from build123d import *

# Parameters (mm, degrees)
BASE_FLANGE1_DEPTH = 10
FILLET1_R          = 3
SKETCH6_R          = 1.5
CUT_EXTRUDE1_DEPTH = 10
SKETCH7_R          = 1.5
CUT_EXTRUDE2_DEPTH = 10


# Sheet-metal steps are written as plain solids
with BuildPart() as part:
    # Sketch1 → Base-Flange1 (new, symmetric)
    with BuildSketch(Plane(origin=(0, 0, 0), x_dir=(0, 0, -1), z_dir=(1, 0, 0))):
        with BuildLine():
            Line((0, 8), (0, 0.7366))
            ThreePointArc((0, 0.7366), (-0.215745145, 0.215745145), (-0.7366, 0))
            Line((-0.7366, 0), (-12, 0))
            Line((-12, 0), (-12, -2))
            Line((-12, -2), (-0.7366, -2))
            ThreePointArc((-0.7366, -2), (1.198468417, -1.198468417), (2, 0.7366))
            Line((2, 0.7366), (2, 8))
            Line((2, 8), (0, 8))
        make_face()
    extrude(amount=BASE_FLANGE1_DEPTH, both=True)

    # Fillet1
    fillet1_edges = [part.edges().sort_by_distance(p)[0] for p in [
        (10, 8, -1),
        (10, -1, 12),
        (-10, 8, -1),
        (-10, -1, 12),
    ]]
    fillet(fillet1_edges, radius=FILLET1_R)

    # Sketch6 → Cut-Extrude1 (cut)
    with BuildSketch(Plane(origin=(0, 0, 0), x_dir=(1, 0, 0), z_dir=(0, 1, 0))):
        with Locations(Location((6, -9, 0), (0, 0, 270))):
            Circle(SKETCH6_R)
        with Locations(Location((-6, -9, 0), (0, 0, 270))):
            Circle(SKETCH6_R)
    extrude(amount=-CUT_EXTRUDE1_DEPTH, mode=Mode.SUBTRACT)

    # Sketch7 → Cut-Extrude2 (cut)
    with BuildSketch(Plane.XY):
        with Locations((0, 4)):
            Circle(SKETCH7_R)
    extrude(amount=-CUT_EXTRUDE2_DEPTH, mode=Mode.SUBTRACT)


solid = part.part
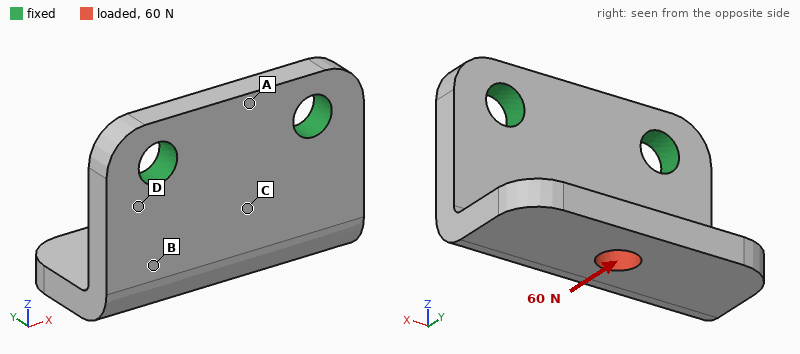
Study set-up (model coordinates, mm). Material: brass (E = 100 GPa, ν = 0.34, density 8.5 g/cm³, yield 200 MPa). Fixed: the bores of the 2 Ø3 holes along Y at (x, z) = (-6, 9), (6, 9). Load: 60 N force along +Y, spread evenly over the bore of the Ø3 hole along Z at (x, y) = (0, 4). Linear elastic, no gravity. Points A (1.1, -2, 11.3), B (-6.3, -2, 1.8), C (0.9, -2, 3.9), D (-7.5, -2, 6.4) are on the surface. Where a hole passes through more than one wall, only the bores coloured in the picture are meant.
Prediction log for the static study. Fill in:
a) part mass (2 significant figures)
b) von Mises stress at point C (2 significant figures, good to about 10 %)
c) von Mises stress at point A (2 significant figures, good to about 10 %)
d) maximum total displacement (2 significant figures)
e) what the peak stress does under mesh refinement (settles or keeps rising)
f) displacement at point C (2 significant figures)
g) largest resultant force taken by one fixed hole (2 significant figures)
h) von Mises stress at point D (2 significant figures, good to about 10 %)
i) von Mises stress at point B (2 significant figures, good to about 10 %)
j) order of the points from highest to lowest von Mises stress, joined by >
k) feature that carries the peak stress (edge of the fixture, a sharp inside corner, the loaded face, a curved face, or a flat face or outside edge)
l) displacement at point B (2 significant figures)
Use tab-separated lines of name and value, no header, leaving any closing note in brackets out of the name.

part mass	6.7 g
von Mises stress at point C	18 MPa
von Mises stress at point A	5.4 MPa
maximum total displacement	22 µm
what the peak stress does under mesh refinement	keeps rising
displacement at point C	4.4 µm
largest resultant force taken by one fixed hole	30 N
von Mises stress at point D	33 MPa
von Mises stress at point B	12 MPa
order of the points from highest to lowest von Mises stress, joined by >	D > C > B > A
feature that carries the peak stress	edge of the fixture
displacement at point B	7.2 µm
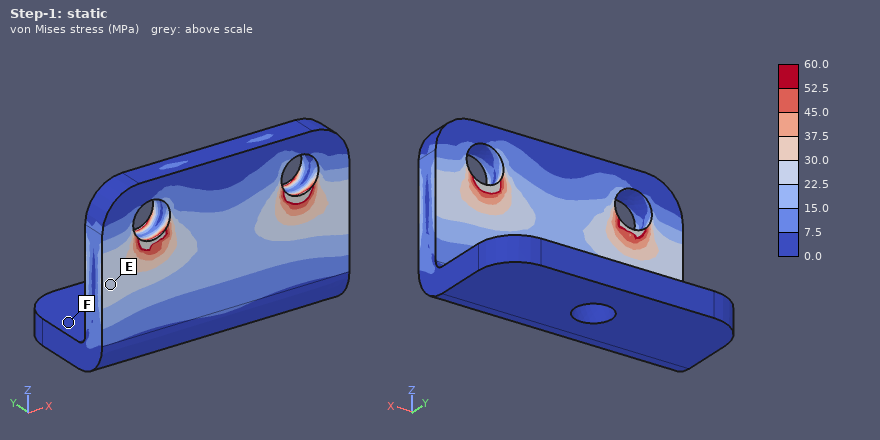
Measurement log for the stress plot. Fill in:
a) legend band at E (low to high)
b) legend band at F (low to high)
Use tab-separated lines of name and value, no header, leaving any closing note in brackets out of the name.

legend band at E	22.5 to 30.0 MPa
legend band at F	0.0 to 7.5 MPa
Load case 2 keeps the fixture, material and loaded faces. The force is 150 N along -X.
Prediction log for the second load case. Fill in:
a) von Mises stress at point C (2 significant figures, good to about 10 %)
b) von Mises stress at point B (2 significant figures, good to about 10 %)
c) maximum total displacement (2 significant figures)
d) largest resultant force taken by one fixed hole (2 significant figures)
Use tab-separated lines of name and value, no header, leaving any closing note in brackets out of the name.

von Mises stress at point C	13 MPa
von Mises stress at point B	17 MPa
maximum total displacement	19 µm
largest resultant force taken by one fixed hole	140 N
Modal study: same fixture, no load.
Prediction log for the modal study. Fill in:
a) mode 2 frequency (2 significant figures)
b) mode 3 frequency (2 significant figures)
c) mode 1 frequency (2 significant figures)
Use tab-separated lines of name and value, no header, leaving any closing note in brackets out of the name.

mode 2 frequency	7900 Hz
mode 3 frequency	13 kHz
mode 1 frequency	4700 Hz
